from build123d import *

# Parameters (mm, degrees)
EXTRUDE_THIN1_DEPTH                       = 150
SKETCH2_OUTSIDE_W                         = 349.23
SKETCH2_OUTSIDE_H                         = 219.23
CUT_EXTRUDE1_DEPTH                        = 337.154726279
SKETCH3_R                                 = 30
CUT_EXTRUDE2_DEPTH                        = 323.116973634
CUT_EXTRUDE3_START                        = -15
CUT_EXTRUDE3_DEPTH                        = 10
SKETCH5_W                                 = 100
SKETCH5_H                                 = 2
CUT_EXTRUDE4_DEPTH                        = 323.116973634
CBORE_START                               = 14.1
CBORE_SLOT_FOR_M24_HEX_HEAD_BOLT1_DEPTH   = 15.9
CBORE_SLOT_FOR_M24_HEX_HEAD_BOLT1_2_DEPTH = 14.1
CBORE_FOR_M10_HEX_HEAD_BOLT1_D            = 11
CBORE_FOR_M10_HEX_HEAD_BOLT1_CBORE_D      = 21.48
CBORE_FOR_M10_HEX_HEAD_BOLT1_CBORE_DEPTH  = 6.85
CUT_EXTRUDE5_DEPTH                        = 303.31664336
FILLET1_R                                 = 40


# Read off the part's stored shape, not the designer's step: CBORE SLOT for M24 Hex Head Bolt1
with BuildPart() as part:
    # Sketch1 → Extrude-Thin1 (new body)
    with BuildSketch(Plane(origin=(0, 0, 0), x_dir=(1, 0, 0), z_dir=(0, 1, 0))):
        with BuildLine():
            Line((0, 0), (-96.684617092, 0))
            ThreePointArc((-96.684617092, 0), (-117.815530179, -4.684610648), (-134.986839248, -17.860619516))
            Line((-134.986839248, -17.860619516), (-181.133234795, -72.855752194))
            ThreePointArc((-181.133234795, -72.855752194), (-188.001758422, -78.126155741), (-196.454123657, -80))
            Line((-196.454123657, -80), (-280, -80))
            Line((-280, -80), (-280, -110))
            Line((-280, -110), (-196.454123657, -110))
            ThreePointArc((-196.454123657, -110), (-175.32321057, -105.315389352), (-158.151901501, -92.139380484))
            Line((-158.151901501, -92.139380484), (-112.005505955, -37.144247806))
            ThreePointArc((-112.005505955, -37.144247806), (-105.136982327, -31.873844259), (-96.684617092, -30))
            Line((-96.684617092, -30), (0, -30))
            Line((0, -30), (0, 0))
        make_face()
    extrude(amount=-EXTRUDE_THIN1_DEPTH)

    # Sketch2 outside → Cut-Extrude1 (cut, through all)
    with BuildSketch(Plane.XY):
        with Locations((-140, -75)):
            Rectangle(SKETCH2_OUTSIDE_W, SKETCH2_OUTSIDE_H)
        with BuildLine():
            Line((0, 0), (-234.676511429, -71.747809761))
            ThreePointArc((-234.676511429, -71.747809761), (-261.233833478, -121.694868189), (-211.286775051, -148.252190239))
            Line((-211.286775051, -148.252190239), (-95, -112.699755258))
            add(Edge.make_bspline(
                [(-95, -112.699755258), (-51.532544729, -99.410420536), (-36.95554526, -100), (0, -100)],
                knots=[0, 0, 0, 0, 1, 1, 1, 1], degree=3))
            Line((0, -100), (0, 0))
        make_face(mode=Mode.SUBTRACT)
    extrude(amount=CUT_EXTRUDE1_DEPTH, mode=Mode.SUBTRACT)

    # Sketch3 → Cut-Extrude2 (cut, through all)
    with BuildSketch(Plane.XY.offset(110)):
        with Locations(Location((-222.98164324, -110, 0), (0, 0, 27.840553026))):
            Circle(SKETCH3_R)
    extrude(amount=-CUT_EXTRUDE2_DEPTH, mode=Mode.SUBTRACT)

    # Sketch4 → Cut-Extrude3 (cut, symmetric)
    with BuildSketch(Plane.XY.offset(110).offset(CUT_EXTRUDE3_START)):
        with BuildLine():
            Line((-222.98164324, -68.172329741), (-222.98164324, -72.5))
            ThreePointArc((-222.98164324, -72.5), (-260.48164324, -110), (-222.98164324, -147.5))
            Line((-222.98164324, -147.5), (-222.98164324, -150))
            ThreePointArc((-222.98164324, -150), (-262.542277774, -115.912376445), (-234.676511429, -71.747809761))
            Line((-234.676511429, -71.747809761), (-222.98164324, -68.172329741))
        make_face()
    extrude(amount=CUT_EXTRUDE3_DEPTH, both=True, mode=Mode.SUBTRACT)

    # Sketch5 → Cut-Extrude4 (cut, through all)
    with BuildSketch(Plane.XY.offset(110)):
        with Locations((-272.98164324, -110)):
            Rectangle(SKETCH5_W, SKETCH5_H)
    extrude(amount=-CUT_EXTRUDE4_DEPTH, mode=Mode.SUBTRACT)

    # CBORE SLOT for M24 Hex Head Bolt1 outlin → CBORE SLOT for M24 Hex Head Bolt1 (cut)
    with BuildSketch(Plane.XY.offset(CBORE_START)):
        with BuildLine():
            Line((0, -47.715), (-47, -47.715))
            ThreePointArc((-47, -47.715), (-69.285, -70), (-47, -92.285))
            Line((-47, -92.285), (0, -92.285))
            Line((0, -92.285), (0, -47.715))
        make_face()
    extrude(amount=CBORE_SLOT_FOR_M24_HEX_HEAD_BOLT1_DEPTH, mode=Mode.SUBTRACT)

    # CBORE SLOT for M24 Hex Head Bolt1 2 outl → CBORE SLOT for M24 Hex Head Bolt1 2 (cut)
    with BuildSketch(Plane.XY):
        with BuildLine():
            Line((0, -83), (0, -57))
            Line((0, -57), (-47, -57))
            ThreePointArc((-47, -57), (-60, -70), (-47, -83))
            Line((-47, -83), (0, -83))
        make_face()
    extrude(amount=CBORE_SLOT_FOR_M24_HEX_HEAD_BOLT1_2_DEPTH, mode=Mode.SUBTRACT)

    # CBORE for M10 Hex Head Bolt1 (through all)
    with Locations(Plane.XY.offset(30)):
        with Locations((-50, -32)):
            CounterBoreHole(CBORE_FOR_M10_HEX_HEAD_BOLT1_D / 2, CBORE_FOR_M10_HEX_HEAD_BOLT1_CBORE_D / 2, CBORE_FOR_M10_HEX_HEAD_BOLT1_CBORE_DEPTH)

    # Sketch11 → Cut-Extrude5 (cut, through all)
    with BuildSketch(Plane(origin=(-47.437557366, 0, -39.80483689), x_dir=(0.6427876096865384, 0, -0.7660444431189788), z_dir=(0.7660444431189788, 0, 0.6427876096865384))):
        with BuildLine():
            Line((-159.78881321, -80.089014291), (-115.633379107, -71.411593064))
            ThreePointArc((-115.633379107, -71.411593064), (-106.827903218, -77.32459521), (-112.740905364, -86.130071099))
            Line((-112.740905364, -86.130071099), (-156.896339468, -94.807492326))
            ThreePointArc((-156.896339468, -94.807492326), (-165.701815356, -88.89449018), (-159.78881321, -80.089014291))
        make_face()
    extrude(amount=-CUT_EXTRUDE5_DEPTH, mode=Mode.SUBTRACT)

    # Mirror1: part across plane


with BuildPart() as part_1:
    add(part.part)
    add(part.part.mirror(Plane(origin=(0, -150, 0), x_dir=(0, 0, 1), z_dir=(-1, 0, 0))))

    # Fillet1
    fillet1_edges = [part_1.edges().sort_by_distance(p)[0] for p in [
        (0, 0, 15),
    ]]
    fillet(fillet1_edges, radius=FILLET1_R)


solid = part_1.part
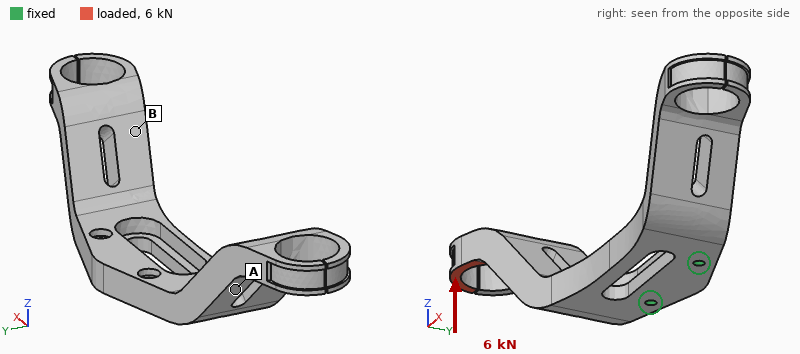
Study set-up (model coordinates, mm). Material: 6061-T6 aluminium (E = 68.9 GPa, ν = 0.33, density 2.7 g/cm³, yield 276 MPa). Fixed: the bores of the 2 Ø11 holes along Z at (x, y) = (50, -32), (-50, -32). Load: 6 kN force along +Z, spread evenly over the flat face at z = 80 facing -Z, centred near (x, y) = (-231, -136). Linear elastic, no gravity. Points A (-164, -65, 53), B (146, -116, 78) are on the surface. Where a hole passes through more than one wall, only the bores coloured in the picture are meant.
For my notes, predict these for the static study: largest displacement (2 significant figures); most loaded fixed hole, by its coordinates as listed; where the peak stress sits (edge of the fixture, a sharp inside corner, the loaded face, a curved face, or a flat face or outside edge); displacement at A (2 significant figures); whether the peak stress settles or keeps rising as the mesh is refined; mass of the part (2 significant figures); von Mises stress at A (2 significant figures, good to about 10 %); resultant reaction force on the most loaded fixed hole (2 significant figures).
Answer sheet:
3.9 mm
(-50, -32)
edge of the fixture
1.2 mm
keeps rising
2.9 kg
51 MPa
10 kN
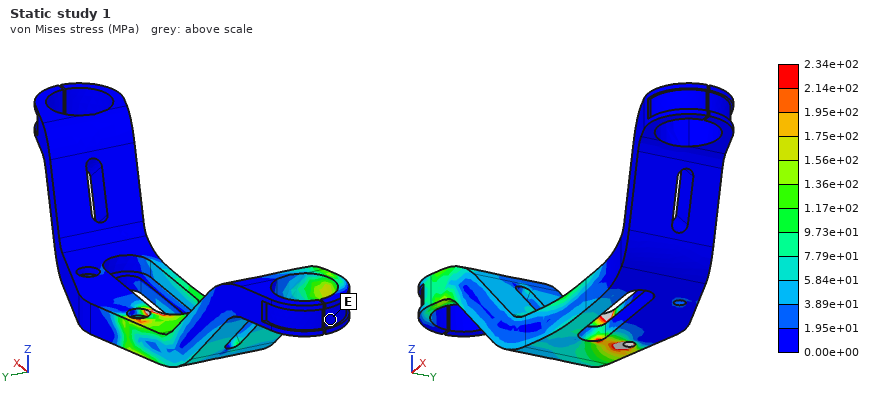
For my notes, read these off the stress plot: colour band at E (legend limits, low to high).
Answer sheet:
0.00e+00 to 1.95e+01 MPa
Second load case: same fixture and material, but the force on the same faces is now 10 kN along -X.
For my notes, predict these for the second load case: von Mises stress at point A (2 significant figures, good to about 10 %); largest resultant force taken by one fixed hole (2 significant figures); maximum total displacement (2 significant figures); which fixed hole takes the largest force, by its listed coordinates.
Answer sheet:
44 MPa
11 kN
2.2 mm
(50, -32)
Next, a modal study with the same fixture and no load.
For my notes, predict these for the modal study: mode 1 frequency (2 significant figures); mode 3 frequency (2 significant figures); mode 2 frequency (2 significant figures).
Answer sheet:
390 Hz
520 Hz
400 Hz
